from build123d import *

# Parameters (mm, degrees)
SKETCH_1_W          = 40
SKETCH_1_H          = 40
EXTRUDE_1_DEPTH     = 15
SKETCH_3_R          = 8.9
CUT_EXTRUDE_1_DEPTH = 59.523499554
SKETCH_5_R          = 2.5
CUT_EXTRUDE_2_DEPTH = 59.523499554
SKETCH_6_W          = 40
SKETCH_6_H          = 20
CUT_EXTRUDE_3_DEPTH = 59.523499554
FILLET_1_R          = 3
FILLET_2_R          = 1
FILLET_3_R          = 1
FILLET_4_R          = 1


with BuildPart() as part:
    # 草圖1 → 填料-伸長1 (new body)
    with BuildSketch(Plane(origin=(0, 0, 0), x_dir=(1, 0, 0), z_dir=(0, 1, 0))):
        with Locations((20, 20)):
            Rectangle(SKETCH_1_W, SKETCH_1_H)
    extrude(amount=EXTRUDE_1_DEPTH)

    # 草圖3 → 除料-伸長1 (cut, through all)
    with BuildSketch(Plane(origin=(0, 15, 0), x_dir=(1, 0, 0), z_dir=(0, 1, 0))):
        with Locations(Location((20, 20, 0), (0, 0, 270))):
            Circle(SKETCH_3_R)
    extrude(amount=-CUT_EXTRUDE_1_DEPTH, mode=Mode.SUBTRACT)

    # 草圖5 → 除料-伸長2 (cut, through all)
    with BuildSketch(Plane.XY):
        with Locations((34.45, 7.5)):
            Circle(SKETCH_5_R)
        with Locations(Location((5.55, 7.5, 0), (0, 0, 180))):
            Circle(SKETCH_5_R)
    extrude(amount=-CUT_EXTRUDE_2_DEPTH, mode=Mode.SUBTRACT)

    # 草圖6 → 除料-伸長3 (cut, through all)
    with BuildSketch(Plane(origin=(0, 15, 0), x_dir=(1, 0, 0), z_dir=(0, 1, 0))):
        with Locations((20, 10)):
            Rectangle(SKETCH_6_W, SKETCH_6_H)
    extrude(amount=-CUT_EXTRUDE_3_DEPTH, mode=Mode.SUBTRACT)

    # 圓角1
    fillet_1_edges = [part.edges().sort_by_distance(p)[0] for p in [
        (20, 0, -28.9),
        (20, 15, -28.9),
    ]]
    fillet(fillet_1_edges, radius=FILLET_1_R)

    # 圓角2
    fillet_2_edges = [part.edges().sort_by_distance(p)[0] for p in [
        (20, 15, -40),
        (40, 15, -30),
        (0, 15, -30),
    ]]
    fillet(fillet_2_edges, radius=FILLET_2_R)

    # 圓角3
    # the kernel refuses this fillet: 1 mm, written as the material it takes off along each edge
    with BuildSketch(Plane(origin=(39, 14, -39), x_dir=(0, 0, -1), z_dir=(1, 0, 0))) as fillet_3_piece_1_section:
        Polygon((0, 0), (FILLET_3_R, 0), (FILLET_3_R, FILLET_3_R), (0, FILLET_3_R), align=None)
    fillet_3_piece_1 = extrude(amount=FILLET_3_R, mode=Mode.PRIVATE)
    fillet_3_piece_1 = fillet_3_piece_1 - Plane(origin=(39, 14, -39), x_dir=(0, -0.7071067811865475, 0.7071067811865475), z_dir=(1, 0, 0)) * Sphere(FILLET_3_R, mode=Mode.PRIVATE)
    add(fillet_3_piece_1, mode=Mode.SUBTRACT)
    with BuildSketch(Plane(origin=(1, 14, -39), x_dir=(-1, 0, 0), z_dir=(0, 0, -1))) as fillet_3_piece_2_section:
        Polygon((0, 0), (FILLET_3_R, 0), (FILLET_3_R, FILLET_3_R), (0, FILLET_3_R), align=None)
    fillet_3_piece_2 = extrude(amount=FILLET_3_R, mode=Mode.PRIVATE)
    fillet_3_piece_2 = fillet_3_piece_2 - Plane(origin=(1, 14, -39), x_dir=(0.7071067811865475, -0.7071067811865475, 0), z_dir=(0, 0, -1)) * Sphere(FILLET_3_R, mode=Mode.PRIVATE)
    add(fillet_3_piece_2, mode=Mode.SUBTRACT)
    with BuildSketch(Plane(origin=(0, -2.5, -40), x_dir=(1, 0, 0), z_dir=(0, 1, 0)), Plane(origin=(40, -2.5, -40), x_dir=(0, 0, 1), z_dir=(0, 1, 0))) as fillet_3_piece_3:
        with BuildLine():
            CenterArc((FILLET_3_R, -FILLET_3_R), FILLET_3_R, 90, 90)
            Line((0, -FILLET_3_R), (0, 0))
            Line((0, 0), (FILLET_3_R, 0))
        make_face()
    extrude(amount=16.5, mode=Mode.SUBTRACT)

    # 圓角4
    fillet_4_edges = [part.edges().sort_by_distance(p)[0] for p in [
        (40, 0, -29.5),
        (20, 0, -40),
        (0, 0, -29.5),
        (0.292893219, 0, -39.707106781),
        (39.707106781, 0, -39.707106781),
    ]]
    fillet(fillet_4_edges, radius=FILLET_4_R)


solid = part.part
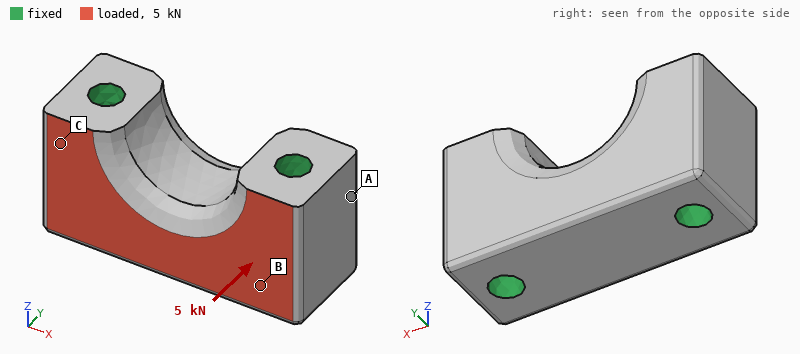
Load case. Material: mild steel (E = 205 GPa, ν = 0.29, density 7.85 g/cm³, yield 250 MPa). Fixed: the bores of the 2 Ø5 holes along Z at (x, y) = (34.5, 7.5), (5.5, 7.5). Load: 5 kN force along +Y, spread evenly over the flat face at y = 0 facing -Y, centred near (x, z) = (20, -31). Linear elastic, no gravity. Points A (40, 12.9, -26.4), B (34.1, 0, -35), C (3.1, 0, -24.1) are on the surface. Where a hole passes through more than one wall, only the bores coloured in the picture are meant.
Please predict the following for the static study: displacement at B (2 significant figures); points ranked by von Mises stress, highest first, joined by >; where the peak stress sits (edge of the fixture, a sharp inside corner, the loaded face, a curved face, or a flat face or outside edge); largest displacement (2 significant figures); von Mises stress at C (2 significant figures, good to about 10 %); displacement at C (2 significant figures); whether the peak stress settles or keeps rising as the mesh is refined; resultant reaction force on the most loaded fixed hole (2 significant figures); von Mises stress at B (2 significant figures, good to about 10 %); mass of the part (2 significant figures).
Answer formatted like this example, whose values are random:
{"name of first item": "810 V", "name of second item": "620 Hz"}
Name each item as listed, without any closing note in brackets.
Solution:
{"displacement at B": "0.37 µm", "points ranked by von Mises stress, highest first, joined by >": "B > C > A", "where the peak stress sits": "edge of the fixture", "largest displacement": "1.2 µm", "von Mises stress at C": "8.4 MPa", "displacement at C": "0.26 µm", "whether the peak stress settles or keeps rising as the mesh is refined": "keeps rising", "resultant reaction force on the most loaded fixed hole": "2.5 kN", "von Mises stress at B": "13 MPa", "mass of the part": "72 g"}
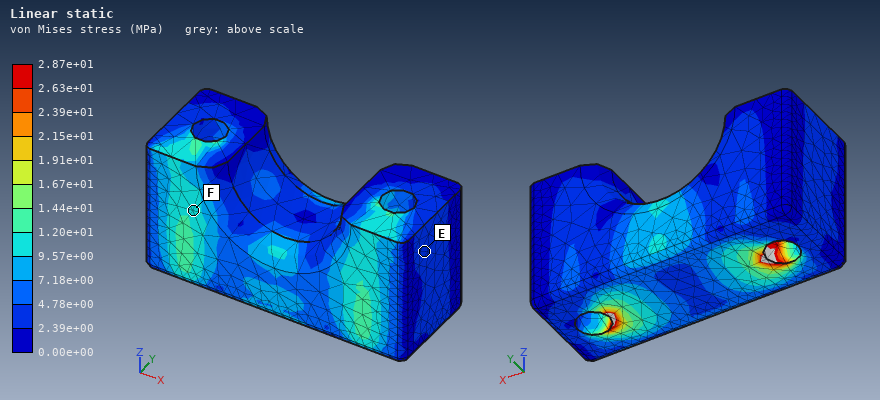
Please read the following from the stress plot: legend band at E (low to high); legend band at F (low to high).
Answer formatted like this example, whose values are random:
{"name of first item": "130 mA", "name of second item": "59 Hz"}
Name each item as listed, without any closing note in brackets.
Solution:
{"legend band at E": "2.39e+00 to 4.78e+00 MPa", "legend band at F": "9.57e+00 to 1.20e+01 MPa"}
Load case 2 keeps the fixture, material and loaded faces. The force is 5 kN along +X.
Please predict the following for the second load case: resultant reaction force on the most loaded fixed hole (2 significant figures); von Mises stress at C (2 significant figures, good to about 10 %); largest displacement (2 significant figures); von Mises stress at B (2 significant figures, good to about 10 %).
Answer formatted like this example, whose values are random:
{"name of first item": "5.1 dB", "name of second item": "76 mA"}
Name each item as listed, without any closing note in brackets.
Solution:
{"resultant reaction force on the most loaded fixed hole": "2.6 kN", "von Mises stress at C": "19 MPa", "largest displacement": "1.3 µm", "von Mises stress at B": "18 MPa"}
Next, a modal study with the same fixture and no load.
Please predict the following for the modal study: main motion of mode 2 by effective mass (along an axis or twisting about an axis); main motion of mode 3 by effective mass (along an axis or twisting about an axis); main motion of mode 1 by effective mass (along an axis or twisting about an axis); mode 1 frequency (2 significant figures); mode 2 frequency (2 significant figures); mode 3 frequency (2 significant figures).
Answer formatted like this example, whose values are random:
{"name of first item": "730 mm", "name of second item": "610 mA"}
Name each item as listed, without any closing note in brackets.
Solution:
{"main motion of mode 2 by effective mass": "along Z", "main motion of mode 3 by effective mass": "twisting about X", "main motion of mode 1 by effective mass": "along Y", "mode 1 frequency": "45 kHz", "mode 2 frequency": "55 kHz", "mode 3 frequency": "67 kHz"}
